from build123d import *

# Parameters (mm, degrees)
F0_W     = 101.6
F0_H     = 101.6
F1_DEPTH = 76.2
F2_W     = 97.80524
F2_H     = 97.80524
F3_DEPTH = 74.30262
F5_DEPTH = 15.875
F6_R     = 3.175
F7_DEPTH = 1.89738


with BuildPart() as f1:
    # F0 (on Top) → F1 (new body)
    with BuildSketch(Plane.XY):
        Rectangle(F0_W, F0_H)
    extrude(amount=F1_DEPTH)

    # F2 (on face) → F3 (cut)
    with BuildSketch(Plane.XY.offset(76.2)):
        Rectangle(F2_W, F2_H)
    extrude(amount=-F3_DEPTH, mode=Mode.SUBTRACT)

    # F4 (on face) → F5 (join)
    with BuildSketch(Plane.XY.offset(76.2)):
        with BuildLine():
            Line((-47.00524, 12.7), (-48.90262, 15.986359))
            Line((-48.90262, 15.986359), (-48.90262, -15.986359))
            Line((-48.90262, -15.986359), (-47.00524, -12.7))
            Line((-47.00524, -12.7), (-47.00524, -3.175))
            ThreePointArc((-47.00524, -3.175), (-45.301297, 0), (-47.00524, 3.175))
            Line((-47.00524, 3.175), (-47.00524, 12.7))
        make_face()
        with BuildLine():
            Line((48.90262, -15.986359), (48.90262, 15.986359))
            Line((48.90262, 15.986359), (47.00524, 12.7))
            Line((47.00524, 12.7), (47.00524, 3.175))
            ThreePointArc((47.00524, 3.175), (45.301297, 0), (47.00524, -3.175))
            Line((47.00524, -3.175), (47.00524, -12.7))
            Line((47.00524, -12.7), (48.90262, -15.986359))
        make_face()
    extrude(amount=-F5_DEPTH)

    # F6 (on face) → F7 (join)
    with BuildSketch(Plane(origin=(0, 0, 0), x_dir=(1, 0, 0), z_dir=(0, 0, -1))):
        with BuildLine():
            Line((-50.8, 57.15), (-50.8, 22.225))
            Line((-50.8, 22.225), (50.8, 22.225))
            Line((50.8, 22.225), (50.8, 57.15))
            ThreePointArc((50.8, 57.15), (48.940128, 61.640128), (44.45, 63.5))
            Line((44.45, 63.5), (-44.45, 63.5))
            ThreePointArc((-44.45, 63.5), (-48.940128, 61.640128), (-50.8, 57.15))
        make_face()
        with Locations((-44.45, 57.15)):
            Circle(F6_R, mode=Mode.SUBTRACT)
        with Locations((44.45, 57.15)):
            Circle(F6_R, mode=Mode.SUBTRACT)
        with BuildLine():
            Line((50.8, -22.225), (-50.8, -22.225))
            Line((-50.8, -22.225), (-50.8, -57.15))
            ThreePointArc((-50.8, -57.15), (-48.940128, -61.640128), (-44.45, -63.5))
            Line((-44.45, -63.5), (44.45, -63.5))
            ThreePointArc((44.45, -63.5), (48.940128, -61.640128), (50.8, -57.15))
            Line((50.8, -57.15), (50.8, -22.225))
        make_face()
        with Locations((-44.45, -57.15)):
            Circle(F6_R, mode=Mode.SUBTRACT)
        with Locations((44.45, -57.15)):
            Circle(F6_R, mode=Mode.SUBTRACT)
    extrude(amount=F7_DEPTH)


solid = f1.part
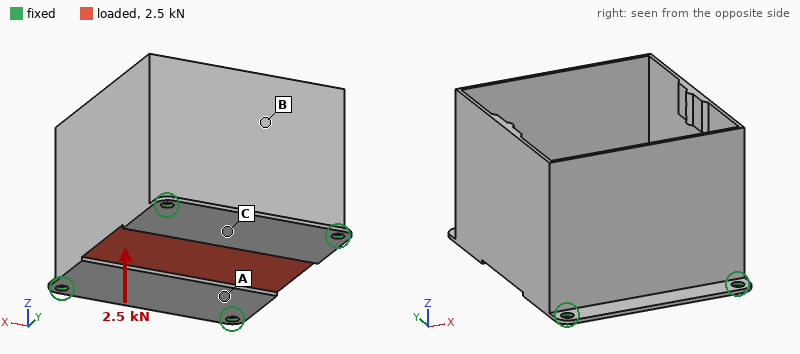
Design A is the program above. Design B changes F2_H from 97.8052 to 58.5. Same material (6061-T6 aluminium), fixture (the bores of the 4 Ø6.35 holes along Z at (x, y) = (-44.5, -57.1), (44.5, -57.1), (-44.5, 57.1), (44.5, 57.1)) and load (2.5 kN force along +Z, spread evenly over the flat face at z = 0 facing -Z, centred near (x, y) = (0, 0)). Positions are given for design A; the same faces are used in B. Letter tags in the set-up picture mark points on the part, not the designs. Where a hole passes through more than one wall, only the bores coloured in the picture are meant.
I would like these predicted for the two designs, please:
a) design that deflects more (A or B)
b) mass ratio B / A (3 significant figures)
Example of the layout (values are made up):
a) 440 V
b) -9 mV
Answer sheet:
a) A
b) 4.06
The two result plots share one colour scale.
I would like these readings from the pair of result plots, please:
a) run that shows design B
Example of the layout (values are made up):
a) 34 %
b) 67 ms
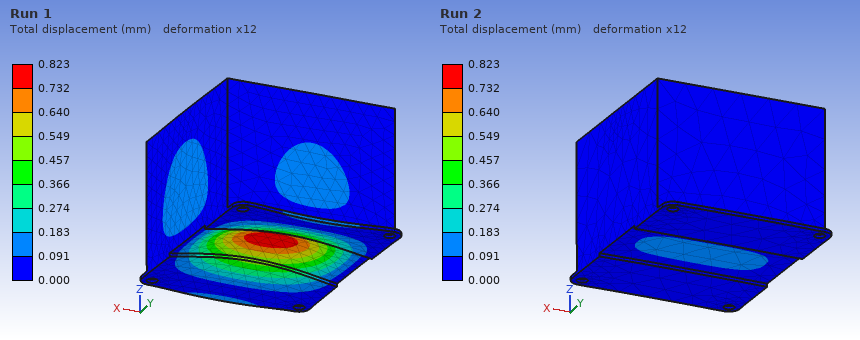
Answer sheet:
a) Run 2
